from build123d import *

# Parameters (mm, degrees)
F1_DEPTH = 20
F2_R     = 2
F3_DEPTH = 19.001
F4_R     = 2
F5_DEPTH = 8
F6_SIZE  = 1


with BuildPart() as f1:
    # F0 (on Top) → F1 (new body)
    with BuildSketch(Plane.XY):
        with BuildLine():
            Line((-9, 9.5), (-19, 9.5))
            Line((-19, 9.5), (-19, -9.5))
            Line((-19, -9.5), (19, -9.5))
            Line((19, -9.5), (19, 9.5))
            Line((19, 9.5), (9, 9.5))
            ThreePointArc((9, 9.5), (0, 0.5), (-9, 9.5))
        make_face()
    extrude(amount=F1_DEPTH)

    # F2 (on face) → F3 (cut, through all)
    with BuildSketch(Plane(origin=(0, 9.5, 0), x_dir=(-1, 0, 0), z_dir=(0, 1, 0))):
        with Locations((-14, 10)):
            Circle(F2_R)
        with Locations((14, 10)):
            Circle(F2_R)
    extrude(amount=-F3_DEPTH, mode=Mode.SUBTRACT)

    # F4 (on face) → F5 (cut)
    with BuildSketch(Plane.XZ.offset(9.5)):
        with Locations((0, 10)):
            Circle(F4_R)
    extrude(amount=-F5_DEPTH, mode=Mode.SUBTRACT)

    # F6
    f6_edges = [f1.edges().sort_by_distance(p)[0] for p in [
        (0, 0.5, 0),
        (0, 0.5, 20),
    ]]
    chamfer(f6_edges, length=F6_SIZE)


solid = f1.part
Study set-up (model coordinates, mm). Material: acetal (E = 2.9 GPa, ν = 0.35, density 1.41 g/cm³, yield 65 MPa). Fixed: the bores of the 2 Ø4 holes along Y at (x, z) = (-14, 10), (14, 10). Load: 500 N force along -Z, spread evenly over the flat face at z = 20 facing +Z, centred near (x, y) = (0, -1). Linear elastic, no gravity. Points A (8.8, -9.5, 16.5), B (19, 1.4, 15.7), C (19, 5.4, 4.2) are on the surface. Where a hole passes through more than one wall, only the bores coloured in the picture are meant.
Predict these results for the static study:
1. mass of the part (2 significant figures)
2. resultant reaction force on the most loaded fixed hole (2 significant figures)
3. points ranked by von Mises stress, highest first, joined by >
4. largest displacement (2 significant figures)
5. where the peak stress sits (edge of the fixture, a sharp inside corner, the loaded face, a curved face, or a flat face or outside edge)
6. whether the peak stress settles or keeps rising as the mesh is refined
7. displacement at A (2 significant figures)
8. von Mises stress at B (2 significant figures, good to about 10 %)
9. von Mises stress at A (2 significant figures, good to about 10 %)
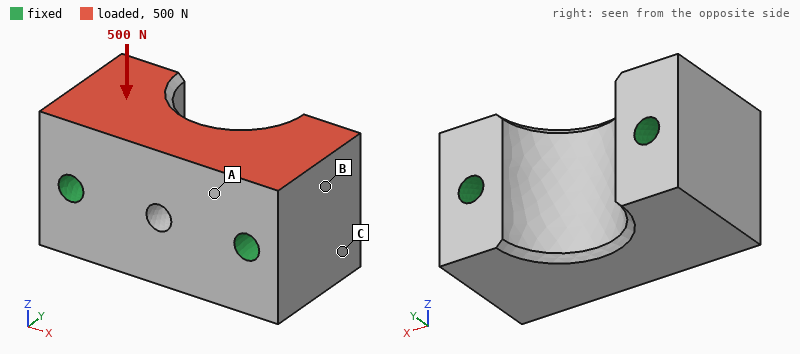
16 g
250 N
A > B > C
9.4 µm
edge of the fixture
keeps rising
5.3 µm
0.62 MPa
1.1 MPa
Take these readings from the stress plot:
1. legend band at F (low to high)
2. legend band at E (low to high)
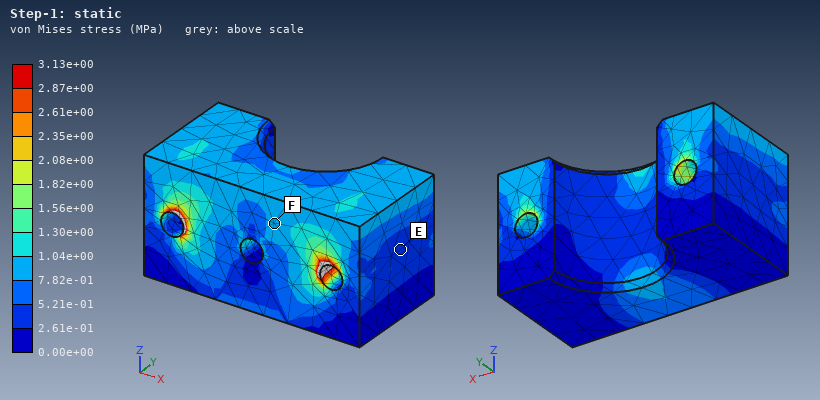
7.82e-01 to 1.04e+00 MPa
2.61e-01 to 5.21e-01 MPa
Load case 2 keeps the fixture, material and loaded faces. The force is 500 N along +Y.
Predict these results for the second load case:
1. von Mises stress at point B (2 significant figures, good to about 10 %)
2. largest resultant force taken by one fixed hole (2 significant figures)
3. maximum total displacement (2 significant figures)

2.3 MPa
250 N
26 µm
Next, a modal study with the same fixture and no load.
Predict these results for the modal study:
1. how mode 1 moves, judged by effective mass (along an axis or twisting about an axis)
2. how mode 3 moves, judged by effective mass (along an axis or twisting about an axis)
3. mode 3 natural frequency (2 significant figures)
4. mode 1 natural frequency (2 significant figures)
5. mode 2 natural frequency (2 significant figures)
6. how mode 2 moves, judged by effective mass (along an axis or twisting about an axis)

along Z
twisting about X
15 kHz
11 kHz
13 kHz
along Y
